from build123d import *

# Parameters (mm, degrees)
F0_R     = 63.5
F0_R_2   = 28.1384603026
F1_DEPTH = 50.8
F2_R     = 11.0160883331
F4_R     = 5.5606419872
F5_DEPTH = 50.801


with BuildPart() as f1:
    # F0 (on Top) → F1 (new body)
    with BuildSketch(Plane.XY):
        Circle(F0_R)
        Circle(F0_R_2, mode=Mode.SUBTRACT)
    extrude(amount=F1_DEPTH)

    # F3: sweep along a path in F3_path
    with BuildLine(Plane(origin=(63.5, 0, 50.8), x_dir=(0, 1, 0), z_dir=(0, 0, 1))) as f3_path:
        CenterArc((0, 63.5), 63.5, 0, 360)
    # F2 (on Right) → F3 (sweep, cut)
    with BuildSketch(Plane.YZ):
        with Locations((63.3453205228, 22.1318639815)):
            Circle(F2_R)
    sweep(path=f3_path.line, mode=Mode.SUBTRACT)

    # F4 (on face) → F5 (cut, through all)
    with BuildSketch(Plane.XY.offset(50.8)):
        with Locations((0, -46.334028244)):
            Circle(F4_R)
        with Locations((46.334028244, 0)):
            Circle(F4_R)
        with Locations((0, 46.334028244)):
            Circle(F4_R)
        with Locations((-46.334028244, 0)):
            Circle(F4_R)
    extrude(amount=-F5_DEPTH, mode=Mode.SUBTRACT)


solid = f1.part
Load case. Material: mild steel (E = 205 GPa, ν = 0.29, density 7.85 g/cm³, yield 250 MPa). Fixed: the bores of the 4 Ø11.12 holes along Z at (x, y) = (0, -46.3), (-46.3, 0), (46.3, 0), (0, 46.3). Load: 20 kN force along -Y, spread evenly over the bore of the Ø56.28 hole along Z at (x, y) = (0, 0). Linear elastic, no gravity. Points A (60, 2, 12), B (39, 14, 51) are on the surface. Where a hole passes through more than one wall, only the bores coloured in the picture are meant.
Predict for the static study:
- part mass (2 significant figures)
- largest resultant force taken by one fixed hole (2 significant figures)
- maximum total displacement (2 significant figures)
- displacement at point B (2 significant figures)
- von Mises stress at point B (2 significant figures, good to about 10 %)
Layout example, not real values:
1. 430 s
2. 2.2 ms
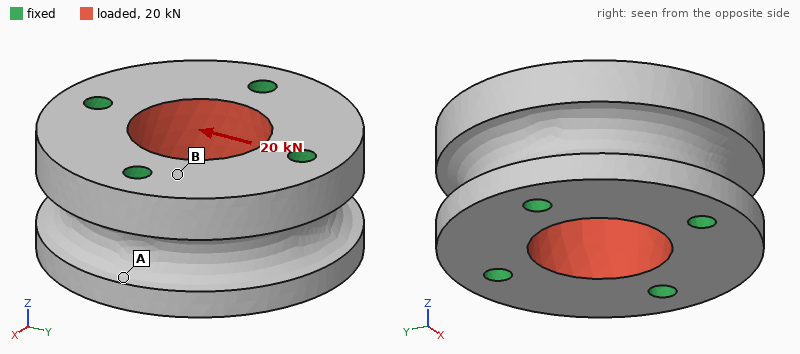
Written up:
1. 3.3 kg
2. 5.1 kN
3. 0.59 µm
4. 0.25 µm
5. 2.2 MPa
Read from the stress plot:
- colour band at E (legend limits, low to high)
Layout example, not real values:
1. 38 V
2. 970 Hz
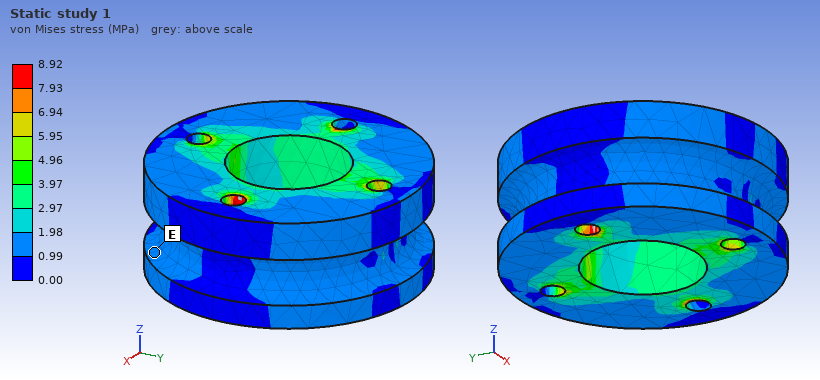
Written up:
1. 0.99 to 1.98 MPa
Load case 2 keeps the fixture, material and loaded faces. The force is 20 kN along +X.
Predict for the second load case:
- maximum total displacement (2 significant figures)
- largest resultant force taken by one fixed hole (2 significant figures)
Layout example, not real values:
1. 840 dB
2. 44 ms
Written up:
1. 0.59 µm
2. 5.1 kN
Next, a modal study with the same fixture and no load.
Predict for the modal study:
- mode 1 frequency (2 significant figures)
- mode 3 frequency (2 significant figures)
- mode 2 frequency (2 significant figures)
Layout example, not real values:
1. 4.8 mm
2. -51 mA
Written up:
1. 16 kHz
2. 17 kHz
3. 17 kHz
